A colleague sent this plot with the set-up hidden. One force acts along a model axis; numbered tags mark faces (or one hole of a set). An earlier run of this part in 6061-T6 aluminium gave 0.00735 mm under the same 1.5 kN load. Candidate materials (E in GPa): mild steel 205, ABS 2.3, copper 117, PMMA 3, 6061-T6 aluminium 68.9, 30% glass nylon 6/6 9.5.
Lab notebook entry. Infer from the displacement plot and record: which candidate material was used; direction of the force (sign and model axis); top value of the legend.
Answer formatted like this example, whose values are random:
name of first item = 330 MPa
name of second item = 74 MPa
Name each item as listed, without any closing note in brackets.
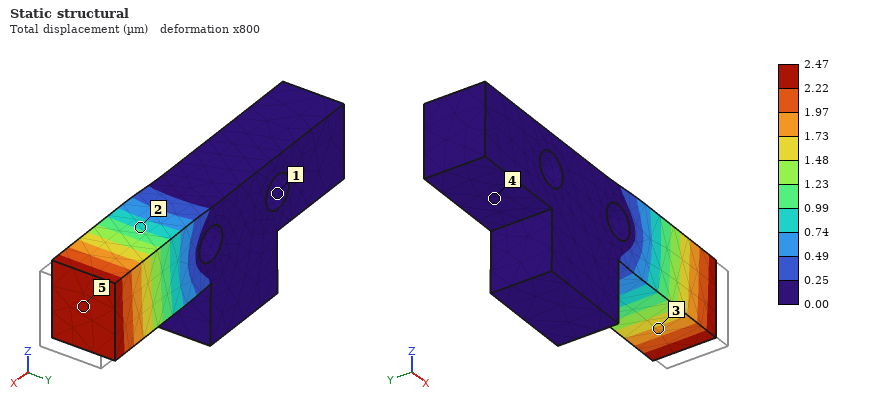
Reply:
which candidate material was used = mild steel
direction of the force = -X
top value of the legend = 2.47 µm
